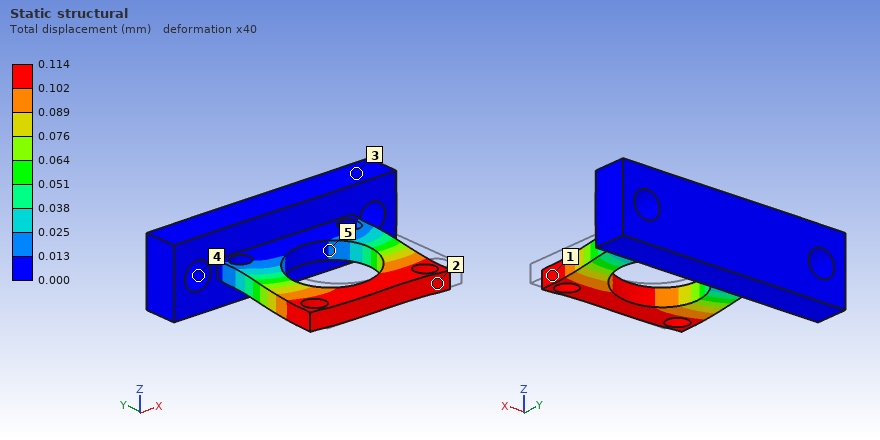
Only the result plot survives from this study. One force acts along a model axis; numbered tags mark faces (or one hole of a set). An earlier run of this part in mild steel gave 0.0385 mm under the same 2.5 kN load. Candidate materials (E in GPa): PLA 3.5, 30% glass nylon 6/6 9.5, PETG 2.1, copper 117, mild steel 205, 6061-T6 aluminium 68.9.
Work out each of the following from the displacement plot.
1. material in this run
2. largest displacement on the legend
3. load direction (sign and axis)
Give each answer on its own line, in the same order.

6061-T6 aluminium
0.114 mm
-X
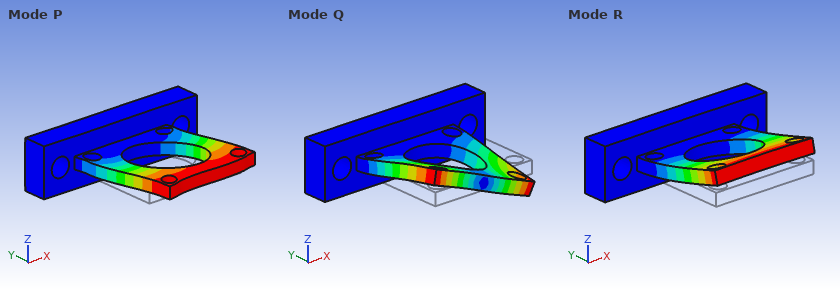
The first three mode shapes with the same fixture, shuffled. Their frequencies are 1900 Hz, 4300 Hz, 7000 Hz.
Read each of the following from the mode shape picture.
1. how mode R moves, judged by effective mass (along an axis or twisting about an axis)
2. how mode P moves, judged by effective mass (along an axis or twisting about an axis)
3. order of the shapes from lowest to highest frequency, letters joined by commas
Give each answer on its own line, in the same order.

along Z
along X
R, Q, P
